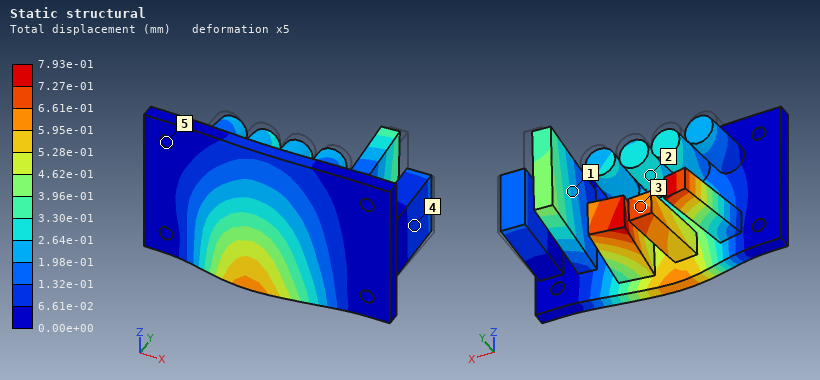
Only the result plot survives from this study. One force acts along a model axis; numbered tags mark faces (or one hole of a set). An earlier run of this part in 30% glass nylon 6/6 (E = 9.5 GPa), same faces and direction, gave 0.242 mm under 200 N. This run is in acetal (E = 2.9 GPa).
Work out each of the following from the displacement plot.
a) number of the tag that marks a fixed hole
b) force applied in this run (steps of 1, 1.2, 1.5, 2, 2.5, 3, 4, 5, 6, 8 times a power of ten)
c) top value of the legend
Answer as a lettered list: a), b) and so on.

a) 5
b) 200 N
c) 7.93e-01 mm
